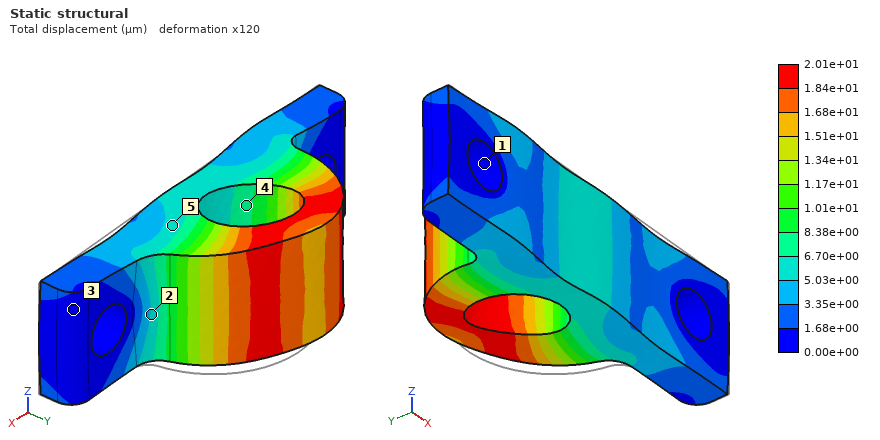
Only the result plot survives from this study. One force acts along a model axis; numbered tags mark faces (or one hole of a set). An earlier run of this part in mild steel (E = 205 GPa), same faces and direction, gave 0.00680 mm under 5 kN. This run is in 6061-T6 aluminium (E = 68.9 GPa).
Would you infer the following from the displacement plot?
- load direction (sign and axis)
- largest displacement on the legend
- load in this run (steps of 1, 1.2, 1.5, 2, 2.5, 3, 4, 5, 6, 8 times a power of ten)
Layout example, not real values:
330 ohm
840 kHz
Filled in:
-X
2.01e+01 µm
5 kN
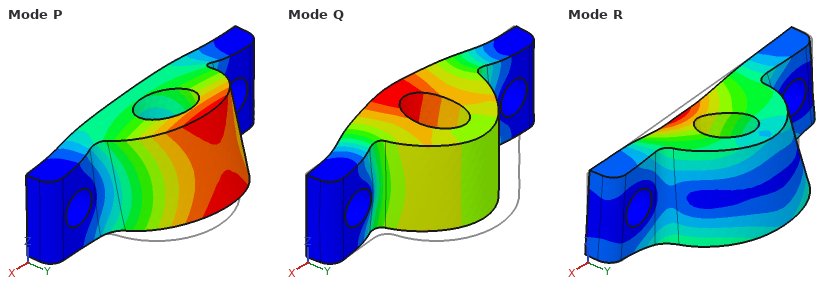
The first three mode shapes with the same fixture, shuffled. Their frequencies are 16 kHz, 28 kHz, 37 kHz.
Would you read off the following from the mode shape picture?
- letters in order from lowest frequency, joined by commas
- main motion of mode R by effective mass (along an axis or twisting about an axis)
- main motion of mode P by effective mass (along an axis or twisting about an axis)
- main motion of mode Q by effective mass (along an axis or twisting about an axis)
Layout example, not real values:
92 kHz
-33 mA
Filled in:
P, Q, R
along Z
along Z
along Y
